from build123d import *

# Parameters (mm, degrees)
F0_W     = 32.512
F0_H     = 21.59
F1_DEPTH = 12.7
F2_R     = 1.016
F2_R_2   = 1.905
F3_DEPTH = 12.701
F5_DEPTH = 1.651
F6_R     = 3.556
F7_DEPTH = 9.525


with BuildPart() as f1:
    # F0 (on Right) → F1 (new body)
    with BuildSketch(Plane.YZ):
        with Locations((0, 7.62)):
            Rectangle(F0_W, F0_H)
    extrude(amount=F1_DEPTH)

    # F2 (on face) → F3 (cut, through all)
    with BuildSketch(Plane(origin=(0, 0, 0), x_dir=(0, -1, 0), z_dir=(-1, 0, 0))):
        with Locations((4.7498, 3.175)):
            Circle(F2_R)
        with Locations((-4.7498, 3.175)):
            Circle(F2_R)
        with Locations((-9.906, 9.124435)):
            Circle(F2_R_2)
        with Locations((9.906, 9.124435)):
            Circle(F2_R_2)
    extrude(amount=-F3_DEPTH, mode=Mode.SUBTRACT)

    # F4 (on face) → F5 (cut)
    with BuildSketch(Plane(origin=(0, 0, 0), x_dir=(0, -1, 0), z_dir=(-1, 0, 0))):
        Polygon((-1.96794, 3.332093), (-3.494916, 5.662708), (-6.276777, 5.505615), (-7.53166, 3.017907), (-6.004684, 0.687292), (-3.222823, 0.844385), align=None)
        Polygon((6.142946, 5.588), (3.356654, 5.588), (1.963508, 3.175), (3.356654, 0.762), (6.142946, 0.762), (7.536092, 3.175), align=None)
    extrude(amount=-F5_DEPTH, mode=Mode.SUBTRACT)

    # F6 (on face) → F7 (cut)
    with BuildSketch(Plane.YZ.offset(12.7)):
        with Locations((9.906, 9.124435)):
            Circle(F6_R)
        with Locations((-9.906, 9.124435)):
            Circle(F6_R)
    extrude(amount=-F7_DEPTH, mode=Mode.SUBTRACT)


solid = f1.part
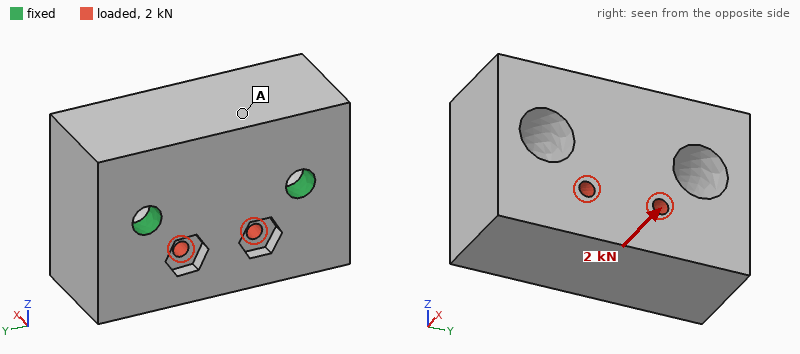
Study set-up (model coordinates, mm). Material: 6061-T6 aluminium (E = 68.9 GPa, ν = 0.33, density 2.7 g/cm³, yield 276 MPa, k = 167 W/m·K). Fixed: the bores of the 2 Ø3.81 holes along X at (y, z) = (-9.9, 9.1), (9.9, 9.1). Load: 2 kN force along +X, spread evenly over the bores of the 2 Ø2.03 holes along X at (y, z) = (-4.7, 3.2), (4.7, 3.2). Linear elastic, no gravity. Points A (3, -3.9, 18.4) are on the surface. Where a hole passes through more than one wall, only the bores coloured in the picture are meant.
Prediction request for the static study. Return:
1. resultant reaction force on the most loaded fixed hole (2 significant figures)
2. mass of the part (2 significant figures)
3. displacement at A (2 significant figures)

1.0 kN
21 g
17 µm
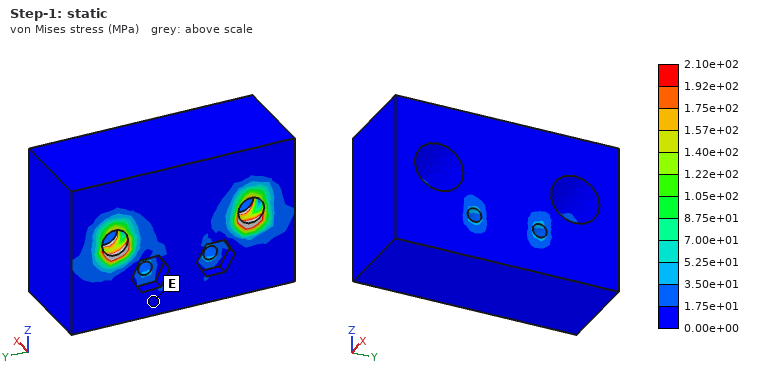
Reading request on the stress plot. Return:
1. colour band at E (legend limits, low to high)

0.00e+00 to 1.75e+01 MPa
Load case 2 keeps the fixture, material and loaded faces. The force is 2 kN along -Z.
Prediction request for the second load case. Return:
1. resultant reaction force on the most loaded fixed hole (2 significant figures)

1.0 kN
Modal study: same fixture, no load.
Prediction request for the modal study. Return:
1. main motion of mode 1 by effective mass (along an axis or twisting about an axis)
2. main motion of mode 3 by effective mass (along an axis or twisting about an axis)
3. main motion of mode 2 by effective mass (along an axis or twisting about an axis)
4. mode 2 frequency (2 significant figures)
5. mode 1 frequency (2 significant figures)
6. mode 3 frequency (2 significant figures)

along Z
twisting about X
along Y
23 kHz
8700 Hz
24 kHz
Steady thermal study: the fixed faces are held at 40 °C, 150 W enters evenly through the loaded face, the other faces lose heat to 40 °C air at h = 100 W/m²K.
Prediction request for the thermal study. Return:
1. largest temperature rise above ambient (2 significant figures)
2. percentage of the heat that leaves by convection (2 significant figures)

52 K
5.8 %
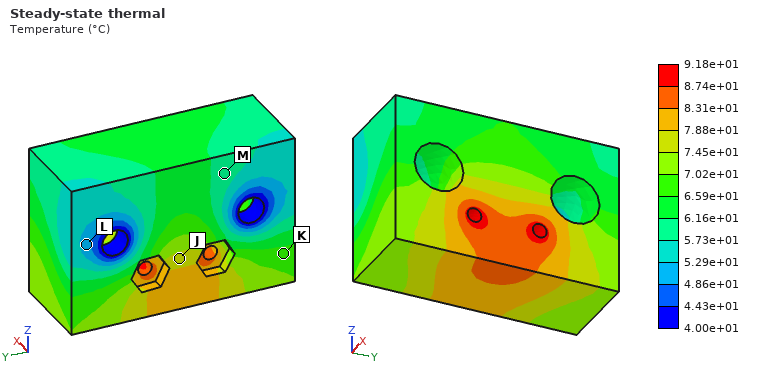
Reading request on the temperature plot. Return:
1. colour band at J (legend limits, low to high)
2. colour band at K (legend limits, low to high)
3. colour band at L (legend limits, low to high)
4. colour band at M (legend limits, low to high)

7.45e+01 to 7.88e+01 °C
6.59e+01 to 7.02e+01 °C
4.86e+01 to 5.29e+01 °C
5.73e+01 to 6.16e+01 °C
